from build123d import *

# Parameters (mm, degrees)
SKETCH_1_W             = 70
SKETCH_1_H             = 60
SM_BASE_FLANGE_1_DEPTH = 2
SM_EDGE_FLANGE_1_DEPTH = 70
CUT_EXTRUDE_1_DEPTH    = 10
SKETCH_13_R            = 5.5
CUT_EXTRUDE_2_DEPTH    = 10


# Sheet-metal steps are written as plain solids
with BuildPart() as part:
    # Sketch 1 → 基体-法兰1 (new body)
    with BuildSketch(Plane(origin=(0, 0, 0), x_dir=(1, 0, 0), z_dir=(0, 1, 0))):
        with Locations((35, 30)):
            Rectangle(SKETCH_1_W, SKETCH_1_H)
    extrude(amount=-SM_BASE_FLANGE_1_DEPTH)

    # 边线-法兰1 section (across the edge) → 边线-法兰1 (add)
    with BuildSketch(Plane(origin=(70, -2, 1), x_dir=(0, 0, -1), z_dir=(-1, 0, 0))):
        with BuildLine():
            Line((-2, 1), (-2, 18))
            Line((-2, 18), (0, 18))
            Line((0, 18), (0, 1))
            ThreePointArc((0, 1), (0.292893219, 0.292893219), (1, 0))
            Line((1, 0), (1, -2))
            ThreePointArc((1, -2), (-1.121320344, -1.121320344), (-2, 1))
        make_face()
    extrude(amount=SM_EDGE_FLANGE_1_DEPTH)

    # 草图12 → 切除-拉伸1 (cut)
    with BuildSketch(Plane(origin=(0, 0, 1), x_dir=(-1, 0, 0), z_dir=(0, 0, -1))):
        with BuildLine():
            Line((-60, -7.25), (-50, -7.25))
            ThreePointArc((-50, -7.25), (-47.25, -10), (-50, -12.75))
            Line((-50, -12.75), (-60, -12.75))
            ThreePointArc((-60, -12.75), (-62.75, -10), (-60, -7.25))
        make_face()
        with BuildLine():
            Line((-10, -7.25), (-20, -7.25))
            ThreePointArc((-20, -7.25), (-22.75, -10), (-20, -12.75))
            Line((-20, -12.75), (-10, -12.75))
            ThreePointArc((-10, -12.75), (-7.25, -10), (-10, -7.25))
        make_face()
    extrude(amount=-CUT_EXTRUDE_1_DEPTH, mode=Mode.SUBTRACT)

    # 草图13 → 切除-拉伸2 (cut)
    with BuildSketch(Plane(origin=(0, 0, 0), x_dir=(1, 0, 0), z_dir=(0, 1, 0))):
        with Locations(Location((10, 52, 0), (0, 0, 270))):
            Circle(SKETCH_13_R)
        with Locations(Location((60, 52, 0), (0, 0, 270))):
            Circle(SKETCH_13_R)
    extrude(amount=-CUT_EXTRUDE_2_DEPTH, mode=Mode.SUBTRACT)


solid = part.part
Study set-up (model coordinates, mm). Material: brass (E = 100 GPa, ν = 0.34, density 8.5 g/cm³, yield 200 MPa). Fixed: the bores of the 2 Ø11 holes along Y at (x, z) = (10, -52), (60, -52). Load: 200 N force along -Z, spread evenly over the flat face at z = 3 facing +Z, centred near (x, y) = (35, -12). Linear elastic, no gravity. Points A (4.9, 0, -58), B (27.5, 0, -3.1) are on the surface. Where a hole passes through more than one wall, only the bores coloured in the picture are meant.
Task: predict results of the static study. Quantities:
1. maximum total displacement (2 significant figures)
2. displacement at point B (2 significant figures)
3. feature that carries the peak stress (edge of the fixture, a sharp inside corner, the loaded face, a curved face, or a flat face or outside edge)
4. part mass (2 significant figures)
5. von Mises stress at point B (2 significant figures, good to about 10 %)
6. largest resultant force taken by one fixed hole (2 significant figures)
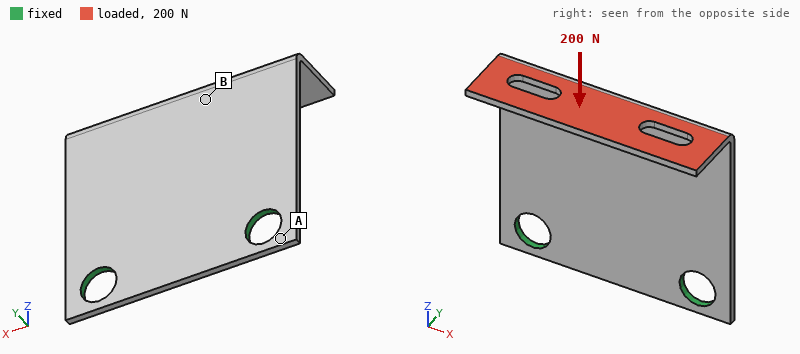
0.76 mm
0.46 mm
a flat face or outside edge
89 g
43 MPa
100 N
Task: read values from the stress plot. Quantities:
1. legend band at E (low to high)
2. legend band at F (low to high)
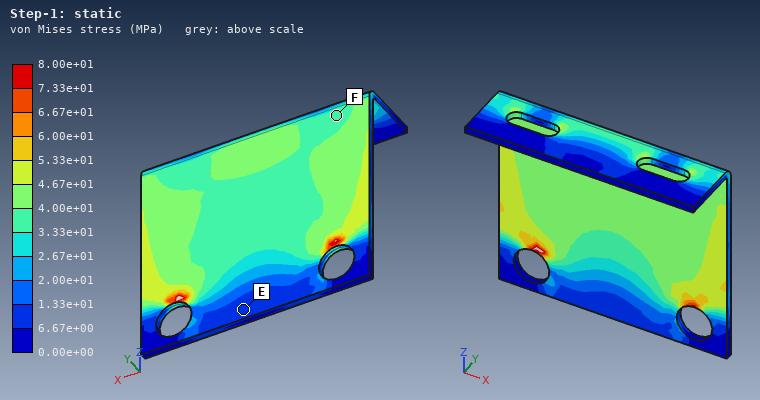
6.67e+00 to 1.33e+01 MPa
3.33e+01 to 4.00e+01 MPa
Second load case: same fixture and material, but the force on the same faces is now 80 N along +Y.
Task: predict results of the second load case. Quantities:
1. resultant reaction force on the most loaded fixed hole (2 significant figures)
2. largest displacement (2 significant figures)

40 N
0.88 mm
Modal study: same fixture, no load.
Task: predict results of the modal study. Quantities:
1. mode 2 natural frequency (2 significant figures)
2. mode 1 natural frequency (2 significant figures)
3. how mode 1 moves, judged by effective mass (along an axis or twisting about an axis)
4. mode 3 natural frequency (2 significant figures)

600 Hz
280 Hz
along Y
1400 Hz
